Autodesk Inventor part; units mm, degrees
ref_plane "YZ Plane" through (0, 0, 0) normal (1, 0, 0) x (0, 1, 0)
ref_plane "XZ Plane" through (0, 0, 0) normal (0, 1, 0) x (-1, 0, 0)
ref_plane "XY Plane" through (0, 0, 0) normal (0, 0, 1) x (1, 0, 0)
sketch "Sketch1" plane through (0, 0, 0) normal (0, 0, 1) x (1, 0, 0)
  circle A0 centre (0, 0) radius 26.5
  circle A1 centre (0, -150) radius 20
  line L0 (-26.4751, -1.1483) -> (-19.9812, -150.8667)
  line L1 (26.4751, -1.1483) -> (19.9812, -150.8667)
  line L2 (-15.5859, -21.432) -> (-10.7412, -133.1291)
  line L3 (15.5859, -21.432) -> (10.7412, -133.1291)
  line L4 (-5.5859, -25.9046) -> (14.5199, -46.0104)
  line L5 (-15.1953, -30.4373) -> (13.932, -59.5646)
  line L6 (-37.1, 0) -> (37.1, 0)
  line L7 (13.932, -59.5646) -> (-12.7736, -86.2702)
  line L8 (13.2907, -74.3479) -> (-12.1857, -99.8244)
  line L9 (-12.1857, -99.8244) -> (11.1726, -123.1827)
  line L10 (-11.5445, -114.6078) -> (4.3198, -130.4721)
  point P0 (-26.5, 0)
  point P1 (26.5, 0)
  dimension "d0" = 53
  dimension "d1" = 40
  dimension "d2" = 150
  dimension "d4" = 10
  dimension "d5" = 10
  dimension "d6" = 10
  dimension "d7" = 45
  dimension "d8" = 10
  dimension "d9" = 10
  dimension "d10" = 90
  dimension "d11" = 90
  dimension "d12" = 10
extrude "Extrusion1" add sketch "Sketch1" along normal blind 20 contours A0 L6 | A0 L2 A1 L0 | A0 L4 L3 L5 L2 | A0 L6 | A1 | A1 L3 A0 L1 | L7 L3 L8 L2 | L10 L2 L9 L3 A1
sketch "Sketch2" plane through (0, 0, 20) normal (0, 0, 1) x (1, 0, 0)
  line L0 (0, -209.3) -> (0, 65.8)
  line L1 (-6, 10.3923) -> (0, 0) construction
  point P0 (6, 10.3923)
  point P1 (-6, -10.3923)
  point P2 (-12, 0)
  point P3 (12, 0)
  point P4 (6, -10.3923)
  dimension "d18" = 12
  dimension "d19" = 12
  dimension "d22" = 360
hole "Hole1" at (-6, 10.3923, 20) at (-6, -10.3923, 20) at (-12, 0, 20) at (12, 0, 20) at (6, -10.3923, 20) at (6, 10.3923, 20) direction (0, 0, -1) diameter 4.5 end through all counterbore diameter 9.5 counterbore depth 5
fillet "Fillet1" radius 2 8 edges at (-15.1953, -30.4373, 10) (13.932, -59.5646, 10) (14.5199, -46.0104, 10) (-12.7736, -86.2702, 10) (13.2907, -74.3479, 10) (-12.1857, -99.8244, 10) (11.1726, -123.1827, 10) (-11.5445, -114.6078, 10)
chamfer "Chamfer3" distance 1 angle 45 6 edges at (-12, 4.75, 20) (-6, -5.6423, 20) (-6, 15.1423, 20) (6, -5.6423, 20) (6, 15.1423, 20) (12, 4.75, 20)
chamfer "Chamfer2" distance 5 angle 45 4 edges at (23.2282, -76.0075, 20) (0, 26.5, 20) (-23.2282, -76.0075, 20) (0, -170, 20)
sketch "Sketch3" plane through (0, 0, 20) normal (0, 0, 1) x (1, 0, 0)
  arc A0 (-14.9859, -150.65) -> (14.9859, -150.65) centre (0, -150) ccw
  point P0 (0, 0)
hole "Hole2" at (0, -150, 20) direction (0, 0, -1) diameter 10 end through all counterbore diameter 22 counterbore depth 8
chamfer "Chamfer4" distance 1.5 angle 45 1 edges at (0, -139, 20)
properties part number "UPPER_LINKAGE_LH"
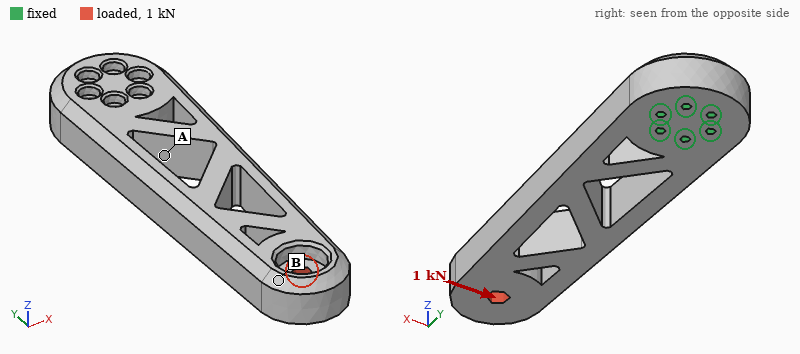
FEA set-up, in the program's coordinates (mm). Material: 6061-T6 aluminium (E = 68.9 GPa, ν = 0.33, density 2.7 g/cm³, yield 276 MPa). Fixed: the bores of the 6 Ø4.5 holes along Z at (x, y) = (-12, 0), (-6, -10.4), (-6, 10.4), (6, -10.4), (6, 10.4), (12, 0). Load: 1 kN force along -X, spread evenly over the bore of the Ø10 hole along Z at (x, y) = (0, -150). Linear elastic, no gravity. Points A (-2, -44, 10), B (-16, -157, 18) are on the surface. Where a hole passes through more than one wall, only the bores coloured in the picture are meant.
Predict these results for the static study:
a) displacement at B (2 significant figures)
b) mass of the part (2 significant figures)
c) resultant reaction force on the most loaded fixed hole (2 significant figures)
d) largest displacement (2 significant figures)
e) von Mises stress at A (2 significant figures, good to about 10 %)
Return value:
0.14 mm
340 g
2.5 kN
0.16 mm
7.4 MPa
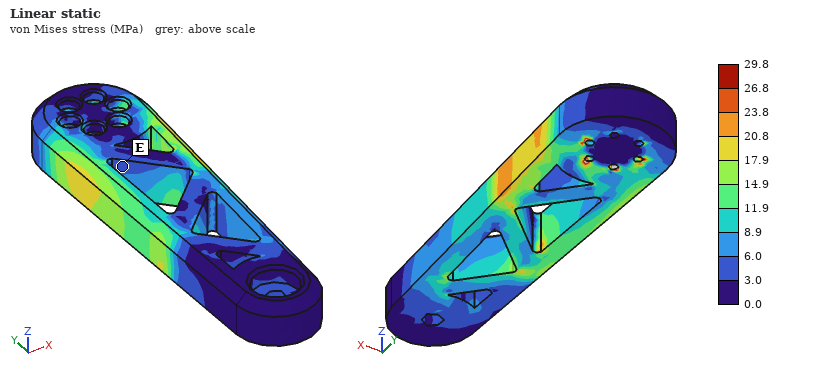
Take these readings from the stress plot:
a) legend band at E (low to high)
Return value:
3.0 to 6.0 MPa
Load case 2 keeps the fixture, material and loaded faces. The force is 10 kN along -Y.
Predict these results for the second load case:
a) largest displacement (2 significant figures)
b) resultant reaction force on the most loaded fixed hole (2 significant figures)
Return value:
0.44 mm
2.5 kN
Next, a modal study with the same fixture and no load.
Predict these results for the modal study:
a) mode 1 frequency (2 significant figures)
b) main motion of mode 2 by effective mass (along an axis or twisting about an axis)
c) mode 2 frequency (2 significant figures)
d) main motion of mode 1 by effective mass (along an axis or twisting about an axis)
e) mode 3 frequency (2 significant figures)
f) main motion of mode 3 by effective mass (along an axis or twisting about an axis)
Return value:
560 Hz
along X
1400 Hz
along Z
2700 Hz
twisting about Y
